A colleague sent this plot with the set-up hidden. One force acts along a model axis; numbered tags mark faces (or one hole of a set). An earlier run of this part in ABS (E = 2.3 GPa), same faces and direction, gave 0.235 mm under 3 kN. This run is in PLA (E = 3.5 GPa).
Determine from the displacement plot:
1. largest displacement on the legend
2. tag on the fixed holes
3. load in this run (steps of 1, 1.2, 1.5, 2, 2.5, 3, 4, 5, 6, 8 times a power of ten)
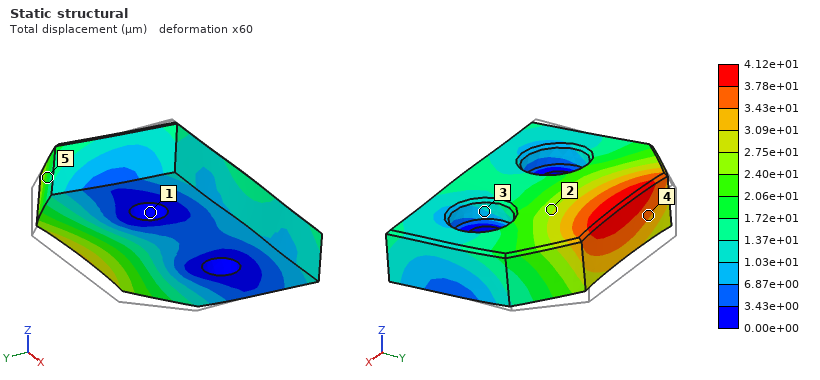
4.12e+01 µm
1
800 N
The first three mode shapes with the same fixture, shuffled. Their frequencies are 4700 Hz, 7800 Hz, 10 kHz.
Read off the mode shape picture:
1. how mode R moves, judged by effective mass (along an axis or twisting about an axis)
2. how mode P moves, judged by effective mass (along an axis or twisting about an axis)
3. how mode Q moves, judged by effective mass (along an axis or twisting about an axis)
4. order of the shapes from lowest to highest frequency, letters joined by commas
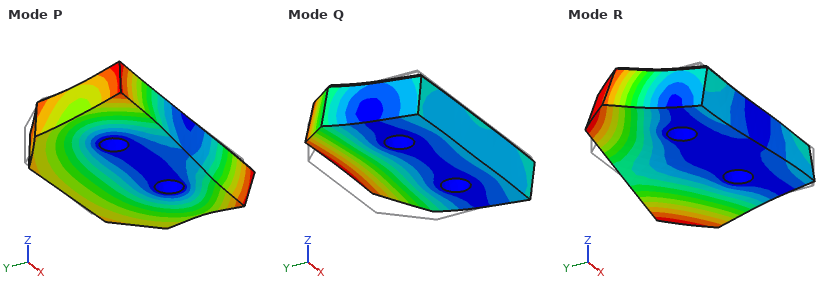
twisting about Y
along X
along Z
Q, R, P
